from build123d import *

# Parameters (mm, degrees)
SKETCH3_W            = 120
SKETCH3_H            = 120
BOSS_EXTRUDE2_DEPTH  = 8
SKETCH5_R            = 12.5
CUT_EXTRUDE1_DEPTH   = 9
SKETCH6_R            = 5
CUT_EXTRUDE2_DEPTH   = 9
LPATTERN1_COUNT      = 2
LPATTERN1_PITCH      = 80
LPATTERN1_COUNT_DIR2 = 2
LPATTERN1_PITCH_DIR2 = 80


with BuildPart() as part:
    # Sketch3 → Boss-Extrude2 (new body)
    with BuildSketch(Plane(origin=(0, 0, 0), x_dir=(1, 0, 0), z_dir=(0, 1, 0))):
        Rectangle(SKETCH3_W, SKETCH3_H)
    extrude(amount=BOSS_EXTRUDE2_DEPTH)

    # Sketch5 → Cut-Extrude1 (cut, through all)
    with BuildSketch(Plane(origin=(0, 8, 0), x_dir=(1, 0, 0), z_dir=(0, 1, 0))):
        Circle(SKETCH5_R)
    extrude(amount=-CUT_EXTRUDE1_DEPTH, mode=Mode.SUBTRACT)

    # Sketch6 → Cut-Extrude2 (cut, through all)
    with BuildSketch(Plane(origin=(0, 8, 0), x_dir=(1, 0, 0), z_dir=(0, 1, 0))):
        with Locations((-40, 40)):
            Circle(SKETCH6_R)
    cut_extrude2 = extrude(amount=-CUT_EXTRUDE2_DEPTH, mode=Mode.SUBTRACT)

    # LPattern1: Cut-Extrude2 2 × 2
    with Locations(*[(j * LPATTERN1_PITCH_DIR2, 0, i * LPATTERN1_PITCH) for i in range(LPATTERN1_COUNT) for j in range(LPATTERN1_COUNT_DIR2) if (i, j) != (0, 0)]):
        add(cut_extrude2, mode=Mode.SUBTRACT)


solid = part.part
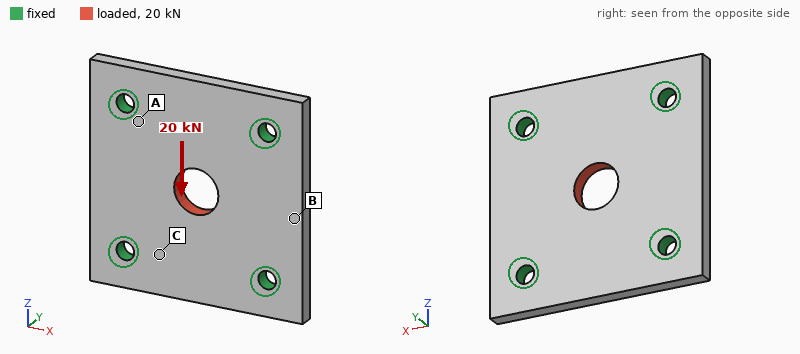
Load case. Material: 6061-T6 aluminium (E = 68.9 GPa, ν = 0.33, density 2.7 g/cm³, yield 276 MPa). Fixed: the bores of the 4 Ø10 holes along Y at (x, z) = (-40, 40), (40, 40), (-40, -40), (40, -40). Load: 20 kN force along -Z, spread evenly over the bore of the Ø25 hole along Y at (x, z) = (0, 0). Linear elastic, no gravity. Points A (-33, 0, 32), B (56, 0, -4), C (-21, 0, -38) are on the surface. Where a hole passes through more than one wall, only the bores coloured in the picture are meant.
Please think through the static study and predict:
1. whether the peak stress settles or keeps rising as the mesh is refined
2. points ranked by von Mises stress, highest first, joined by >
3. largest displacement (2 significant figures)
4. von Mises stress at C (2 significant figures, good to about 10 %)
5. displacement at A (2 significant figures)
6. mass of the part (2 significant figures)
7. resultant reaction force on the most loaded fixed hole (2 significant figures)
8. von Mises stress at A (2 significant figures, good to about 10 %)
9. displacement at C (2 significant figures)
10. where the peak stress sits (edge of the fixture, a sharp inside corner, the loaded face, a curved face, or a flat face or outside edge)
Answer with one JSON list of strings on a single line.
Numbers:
["keeps rising", "A > C > B", "22 µm", "18 MPa", "3.6 µm", "290 g", "5.4 kN", "31 MPa", "9.4 µm", "edge of the fixture"]
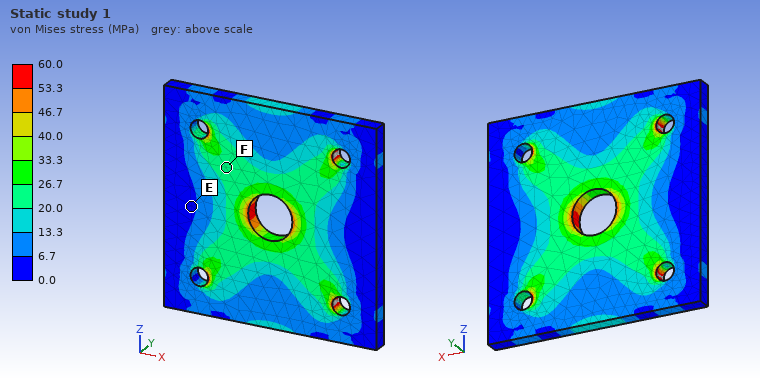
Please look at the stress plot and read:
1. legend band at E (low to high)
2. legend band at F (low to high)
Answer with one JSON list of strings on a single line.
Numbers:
["0.0 to 6.7 MPa", "20.0 to 26.7 MPa"]
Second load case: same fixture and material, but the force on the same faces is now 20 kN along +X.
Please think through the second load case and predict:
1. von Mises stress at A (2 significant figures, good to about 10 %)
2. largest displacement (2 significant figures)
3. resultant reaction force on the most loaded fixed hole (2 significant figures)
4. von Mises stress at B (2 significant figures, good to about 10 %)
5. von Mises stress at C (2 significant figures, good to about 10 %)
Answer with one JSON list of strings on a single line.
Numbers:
["31 MPa", "22 µm", "5.4 kN", "13 MPa", "16 MPa"]
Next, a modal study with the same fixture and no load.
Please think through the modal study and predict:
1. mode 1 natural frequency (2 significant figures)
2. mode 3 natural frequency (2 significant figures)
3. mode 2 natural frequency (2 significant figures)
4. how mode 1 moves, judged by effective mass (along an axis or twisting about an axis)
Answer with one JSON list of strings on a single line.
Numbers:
["5000 Hz", "6700 Hz", "6600 Hz", "along Y"]
